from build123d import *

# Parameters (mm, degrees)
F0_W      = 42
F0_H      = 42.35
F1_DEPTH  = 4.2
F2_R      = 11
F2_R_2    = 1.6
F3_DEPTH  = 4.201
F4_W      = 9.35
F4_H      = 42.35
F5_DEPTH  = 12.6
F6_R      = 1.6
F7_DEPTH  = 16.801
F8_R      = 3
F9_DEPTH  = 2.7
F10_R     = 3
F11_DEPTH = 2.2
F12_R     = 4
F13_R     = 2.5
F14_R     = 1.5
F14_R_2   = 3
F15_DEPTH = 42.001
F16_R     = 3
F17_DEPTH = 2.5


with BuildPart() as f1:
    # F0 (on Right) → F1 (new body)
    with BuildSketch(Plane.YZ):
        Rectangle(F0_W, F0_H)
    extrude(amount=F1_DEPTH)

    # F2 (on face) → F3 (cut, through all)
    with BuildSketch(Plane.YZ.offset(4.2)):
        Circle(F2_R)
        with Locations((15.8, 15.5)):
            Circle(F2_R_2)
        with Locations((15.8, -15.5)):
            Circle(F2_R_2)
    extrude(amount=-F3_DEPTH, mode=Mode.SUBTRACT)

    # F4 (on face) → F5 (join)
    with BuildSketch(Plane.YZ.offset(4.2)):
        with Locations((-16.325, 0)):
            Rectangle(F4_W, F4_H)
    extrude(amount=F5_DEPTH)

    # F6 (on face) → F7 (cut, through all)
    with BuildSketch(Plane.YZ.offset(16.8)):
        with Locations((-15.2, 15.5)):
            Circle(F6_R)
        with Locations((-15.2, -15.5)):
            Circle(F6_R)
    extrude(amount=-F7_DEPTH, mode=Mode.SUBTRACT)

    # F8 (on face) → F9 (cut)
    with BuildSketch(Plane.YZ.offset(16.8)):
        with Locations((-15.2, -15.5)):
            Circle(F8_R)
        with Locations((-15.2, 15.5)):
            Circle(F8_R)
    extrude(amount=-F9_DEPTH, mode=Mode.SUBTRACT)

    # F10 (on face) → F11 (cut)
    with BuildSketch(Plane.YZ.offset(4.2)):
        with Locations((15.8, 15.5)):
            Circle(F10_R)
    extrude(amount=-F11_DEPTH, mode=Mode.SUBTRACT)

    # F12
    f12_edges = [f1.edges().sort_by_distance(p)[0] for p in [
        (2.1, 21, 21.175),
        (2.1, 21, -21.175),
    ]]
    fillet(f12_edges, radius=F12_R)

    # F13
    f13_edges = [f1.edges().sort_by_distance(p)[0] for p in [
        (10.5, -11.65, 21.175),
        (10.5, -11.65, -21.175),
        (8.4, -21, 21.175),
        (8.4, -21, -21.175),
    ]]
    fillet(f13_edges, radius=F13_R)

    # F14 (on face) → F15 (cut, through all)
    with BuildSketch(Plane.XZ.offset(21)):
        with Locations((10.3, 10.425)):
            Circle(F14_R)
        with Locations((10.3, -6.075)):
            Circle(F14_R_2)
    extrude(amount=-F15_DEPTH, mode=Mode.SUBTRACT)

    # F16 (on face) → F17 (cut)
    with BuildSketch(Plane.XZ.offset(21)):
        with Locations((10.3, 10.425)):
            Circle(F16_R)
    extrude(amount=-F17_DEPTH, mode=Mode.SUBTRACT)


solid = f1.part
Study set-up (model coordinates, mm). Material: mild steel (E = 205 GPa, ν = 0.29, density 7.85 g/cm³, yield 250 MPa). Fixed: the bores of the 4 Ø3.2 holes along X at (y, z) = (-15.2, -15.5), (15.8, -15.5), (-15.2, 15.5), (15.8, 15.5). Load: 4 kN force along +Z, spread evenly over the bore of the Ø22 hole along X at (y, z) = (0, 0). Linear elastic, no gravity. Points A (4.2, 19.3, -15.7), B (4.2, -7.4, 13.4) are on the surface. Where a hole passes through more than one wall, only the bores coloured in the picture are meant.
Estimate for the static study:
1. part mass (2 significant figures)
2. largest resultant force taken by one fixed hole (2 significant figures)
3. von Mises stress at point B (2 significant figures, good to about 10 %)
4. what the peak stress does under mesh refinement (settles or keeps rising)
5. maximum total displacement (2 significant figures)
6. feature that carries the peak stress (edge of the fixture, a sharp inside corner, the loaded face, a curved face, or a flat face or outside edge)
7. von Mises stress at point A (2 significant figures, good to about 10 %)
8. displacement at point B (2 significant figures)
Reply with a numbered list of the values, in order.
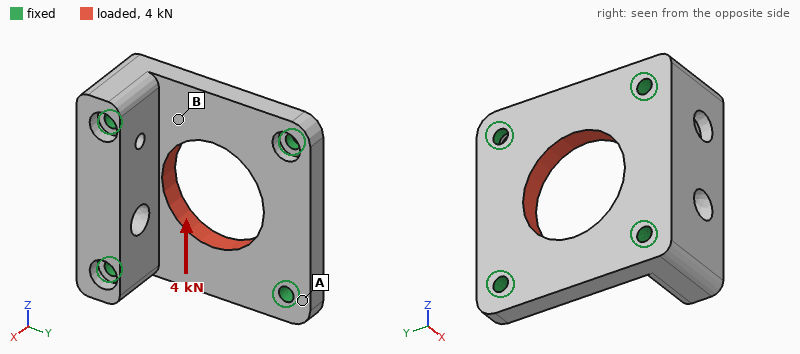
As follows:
1. 78 g
2. 1.1 kN
3. 23 MPa
4. keeps rising
5. 3.2 µm
6. edge of the fixture
7. 8.8 MPa
8. 1.6 µm
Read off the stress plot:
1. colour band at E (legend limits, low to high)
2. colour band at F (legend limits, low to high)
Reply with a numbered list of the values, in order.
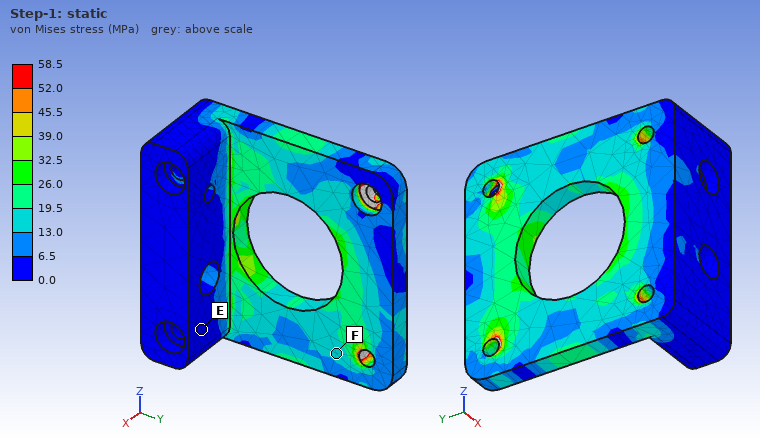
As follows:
1. 0.0 to 6.5 MPa
2. 13.0 to 19.5 MPa
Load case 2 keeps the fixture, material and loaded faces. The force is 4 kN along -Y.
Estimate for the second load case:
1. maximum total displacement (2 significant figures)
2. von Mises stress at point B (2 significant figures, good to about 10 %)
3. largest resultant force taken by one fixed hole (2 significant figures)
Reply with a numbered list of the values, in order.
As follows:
1. 3.6 µm
2. 23 MPa
3. 1.2 kN
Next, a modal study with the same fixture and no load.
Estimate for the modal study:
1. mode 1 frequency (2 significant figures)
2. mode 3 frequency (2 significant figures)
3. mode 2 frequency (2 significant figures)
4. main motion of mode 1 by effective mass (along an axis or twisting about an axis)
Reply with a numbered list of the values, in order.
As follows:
1. 19 kHz
2. 24 kHz
3. 21 kHz
4. along X
